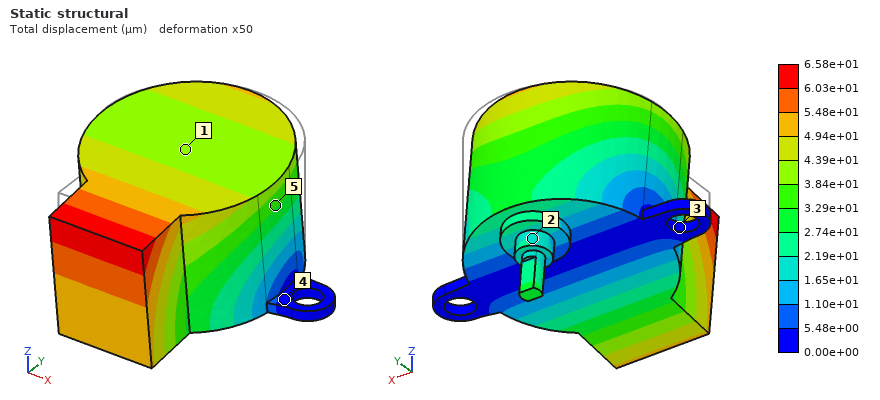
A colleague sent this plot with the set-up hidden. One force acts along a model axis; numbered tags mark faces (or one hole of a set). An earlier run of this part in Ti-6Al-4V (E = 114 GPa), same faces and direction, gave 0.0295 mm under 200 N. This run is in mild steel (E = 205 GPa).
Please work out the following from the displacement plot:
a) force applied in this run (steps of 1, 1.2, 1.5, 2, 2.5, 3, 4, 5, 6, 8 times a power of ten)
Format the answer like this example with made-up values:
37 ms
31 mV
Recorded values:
800 N
